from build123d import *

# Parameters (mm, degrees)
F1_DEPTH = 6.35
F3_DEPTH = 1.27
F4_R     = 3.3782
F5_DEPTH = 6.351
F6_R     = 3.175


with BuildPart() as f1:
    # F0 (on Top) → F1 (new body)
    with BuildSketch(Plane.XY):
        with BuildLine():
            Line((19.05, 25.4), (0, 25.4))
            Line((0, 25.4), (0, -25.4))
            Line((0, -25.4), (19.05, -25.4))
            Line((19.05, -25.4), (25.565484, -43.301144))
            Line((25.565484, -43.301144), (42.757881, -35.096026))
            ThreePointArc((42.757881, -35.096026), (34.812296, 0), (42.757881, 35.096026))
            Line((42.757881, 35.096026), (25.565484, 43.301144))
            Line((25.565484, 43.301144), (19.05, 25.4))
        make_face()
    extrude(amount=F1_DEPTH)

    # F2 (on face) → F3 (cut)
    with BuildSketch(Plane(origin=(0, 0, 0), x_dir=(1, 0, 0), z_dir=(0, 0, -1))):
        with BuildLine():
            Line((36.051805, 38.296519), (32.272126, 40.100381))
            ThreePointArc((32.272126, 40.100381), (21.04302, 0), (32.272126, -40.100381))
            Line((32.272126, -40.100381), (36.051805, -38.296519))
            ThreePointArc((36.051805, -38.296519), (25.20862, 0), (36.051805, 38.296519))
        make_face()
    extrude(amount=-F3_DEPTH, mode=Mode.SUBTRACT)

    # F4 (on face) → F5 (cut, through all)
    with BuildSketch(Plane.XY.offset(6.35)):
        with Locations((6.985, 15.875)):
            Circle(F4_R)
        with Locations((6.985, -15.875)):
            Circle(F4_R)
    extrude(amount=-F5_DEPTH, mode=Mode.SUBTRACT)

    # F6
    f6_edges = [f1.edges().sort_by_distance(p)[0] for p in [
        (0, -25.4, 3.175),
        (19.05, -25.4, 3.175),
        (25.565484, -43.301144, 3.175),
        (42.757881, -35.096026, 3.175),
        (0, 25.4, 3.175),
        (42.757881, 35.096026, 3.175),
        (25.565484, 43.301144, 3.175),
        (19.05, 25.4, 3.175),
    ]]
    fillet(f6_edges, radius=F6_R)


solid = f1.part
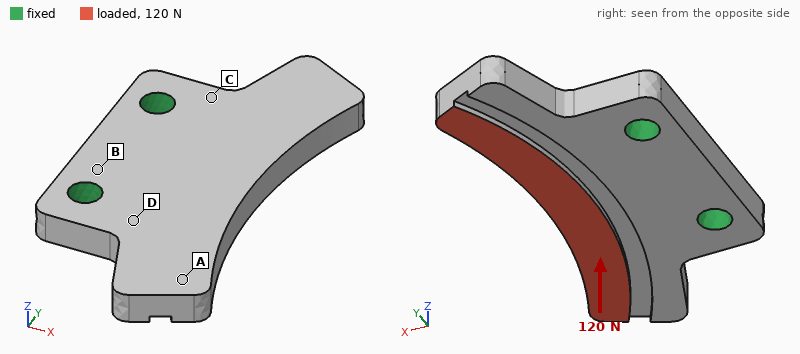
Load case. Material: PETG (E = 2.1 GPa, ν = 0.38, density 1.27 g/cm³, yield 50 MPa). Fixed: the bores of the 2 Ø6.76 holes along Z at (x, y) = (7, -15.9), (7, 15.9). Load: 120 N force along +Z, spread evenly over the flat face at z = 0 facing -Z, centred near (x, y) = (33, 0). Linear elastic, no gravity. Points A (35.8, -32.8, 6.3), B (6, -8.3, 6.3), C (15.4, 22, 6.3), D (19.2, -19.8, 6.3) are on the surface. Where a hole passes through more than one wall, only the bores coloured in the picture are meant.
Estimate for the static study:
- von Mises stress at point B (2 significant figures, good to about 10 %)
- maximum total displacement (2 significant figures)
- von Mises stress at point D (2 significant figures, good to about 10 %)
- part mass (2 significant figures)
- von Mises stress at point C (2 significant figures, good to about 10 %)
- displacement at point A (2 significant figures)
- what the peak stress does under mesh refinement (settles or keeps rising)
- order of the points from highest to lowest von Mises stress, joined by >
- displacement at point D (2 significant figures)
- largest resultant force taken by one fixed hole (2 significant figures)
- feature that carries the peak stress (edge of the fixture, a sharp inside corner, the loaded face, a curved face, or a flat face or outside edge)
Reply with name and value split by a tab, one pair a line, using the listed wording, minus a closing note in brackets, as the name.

von Mises stress at point B	2.7 MPa
maximum total displacement	0.49 mm
von Mises stress at point D	5.0 MPa
part mass	18 g
von Mises stress at point C	6.6 MPa
displacement at point A	0.38 mm
what the peak stress does under mesh refinement	keeps rising
order of the points from highest to lowest von Mises stress, joined by >	C > D > B > A
displacement at point D	0.087 mm
largest resultant force taken by one fixed hole	60 N
feature that carries the peak stress	edge of the fixture
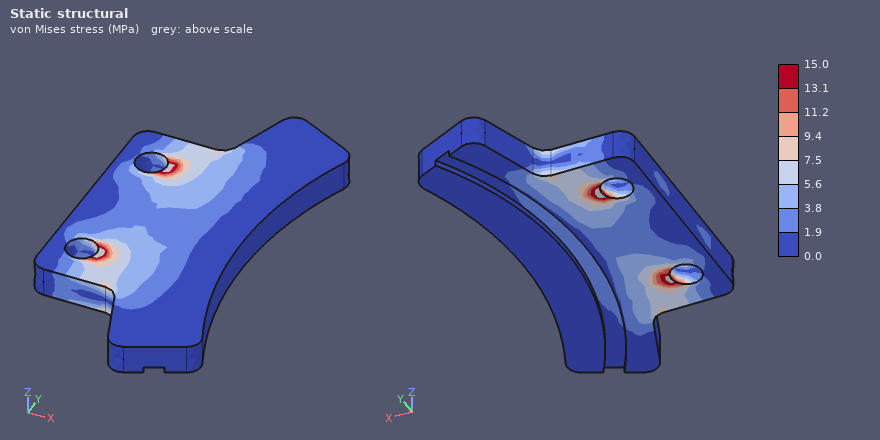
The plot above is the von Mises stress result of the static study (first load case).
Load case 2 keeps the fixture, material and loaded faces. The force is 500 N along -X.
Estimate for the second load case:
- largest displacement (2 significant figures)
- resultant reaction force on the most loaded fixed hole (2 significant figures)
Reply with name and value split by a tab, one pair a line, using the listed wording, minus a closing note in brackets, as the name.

largest displacement	0.41 mm
resultant reaction force on the most loaded fixed hole	250 N
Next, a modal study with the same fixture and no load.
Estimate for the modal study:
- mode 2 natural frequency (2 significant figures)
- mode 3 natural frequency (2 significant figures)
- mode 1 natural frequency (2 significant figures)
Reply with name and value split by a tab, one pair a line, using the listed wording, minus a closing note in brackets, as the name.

mode 2 natural frequency	1100 Hz
mode 3 natural frequency	2000 Hz
mode 1 natural frequency	1100 Hz
